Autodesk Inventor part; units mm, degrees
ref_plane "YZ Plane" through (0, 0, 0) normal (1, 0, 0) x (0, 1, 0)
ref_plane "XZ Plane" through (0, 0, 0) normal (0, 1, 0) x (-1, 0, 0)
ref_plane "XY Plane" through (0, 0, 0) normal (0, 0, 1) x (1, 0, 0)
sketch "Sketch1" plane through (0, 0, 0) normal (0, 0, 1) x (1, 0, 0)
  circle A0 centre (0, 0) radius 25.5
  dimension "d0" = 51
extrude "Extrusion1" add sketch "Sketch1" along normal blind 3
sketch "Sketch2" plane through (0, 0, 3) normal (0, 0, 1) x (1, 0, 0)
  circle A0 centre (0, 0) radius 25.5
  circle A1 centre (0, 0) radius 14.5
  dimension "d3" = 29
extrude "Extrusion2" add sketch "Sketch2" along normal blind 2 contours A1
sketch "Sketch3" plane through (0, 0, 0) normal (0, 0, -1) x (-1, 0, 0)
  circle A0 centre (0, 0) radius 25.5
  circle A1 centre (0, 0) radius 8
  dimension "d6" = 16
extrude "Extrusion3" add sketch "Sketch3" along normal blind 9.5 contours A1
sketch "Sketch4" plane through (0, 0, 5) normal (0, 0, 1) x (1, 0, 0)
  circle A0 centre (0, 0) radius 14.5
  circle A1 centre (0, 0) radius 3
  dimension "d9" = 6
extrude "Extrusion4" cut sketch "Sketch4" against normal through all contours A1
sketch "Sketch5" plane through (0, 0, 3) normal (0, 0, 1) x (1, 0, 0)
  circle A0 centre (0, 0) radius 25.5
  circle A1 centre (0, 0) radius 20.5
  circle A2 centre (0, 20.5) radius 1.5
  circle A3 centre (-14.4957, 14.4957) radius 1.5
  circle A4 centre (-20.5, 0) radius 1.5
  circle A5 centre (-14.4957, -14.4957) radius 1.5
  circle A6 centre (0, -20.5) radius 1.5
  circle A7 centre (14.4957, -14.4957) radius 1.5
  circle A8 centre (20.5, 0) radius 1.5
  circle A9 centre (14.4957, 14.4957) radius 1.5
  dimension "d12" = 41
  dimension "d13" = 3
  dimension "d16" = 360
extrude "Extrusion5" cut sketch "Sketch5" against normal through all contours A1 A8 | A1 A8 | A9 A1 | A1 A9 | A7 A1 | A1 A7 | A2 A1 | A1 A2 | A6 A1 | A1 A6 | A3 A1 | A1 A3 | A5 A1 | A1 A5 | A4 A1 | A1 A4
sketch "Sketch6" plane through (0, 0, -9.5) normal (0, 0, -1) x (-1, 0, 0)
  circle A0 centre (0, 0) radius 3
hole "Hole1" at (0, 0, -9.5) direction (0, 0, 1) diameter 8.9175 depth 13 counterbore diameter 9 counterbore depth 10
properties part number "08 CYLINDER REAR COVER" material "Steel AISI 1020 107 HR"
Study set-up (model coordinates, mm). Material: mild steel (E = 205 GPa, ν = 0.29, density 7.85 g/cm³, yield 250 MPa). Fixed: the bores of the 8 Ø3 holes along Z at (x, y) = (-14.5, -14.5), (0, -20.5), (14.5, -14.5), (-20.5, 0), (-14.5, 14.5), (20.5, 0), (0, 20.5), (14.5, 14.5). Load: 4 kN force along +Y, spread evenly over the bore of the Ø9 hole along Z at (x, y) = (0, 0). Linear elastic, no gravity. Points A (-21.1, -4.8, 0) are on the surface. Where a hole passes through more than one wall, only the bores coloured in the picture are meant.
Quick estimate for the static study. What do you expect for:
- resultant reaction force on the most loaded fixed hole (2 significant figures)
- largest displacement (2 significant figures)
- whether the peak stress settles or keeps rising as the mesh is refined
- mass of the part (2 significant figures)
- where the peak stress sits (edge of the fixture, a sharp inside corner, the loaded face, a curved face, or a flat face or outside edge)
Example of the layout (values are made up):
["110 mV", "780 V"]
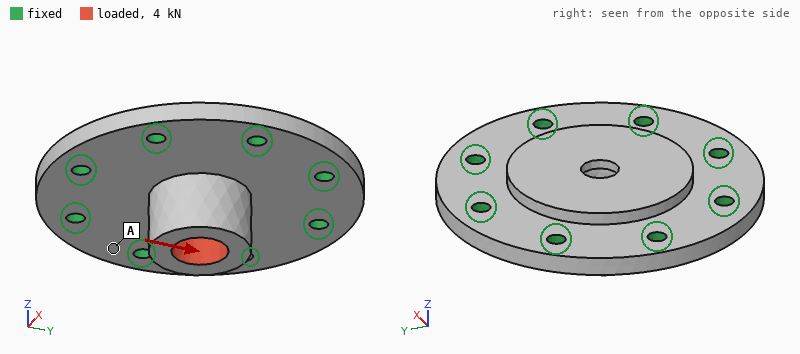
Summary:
["820 N", "15 µm", "keeps rising", "65 g", "edge of the fixture"]
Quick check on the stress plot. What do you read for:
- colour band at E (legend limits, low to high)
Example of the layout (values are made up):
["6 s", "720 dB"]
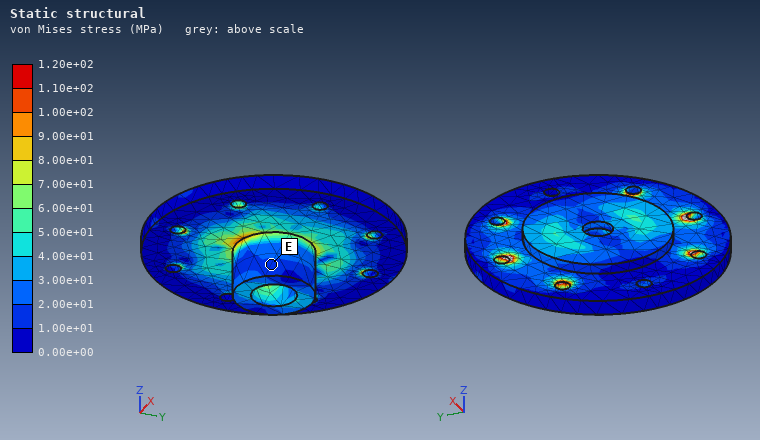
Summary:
["1.00e+01 to 2.00e+01 MPa"]
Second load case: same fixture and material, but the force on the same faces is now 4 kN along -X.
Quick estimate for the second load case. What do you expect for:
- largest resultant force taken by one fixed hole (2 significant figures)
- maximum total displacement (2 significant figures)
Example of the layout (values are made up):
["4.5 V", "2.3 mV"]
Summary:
["820 N", "15 µm"]
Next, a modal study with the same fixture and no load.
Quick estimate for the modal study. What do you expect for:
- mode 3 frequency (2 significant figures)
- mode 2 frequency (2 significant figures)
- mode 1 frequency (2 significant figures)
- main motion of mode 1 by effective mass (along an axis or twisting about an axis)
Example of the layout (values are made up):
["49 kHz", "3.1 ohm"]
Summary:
["24 kHz", "24 kHz", "17 kHz", "along Z"]
